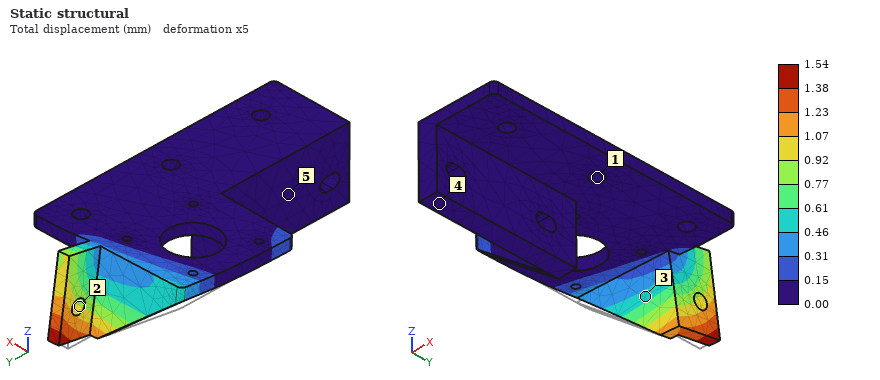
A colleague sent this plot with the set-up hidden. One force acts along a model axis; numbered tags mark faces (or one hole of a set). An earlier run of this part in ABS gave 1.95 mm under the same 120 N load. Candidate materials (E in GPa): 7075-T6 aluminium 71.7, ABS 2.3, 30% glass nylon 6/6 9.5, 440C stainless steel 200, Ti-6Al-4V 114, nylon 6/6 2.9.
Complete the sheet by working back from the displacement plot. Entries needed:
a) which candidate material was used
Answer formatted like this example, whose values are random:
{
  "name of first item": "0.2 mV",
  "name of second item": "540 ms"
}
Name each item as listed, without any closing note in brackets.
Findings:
{
  "which candidate material was used": "nylon 6/6"
}
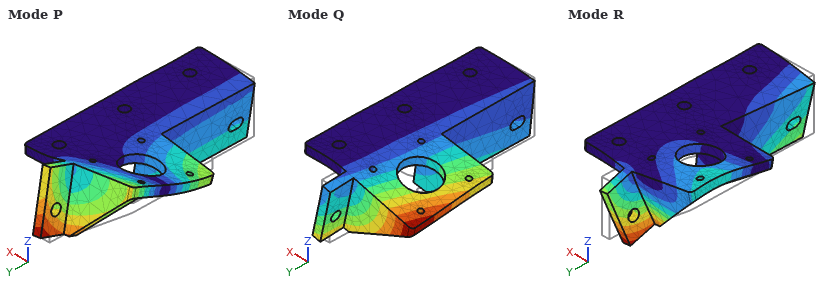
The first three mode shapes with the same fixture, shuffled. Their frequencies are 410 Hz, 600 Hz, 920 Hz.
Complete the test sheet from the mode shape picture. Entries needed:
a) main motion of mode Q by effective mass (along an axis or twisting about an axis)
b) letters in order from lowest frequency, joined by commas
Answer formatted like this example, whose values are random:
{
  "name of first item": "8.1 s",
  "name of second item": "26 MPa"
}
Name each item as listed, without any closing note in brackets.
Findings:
{
  "main motion of mode Q by effective mass": "along Z",
  "letters in order from lowest frequency, joined by commas": "Q, P, R"
}
